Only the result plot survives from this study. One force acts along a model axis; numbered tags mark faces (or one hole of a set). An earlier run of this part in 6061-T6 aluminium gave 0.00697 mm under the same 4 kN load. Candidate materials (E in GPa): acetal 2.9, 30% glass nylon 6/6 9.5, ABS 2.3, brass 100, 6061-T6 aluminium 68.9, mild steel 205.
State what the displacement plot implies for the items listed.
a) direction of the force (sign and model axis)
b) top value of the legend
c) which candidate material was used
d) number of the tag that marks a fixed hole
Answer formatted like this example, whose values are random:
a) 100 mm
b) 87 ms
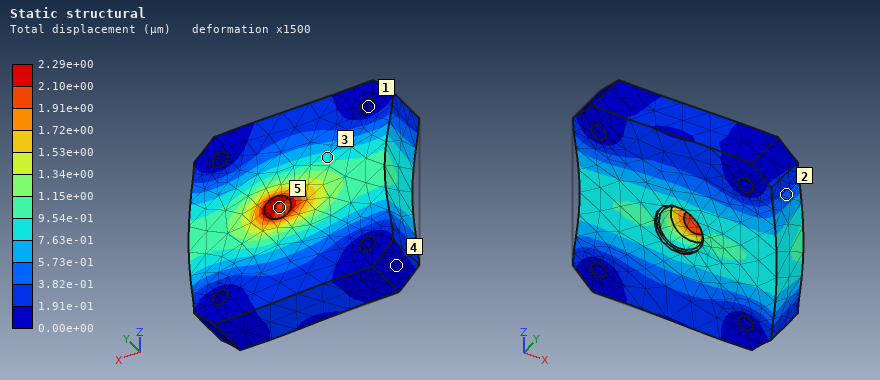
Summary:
a) +X
b) 2.29e+00 µm
c) mild steel
d) 1
